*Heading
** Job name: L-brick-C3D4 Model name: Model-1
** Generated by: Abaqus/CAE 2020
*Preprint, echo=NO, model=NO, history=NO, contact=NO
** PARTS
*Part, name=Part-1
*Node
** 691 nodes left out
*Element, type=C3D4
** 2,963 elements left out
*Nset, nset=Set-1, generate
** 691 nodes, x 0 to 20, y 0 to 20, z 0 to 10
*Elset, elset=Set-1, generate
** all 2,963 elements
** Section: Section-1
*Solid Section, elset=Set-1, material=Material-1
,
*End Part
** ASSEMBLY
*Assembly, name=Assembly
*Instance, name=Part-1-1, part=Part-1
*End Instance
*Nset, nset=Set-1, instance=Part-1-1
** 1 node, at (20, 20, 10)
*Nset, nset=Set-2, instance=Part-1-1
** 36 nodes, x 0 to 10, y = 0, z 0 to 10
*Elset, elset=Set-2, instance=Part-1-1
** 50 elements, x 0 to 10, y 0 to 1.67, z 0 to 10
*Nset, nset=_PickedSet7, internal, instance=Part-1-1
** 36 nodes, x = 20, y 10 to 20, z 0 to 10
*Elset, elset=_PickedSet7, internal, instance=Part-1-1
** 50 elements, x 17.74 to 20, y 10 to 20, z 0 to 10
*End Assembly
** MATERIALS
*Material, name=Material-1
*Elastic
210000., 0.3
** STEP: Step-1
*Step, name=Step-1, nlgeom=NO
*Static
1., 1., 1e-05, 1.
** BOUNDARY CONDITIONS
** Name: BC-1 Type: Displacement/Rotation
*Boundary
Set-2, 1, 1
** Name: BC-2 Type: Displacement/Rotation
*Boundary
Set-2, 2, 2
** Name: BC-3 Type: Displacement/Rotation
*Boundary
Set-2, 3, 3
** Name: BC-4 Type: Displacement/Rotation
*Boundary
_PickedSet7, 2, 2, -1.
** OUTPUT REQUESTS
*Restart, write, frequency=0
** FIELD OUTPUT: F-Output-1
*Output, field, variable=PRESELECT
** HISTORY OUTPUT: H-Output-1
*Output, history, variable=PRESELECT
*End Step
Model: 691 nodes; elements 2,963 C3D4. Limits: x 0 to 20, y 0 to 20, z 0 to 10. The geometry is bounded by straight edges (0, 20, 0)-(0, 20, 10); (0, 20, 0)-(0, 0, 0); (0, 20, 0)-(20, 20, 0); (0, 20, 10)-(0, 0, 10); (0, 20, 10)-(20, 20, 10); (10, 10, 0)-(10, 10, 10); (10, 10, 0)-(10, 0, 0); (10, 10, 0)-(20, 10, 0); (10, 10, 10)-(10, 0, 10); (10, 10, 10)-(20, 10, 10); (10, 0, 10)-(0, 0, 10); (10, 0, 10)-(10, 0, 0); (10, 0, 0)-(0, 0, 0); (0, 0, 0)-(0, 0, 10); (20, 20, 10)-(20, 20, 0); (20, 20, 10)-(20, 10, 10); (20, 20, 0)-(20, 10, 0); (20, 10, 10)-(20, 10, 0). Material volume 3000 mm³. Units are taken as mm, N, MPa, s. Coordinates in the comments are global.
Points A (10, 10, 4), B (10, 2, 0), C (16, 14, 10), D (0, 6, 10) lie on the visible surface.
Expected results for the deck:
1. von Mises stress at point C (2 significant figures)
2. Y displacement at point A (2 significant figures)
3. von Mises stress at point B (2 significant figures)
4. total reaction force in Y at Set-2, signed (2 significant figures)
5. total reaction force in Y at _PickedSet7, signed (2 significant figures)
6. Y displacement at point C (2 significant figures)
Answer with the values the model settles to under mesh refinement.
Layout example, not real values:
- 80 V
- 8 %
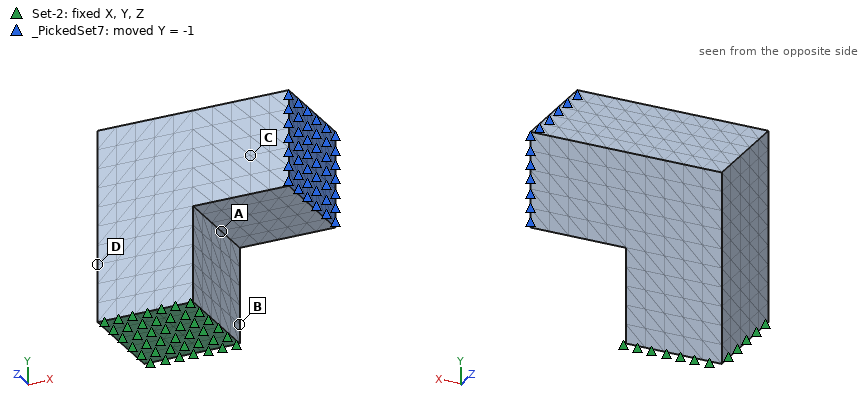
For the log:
- 1300 MPa
- -0.22 mm
- 3900 MPa
- 44000 N
- -44000 N
- -0.69 mm
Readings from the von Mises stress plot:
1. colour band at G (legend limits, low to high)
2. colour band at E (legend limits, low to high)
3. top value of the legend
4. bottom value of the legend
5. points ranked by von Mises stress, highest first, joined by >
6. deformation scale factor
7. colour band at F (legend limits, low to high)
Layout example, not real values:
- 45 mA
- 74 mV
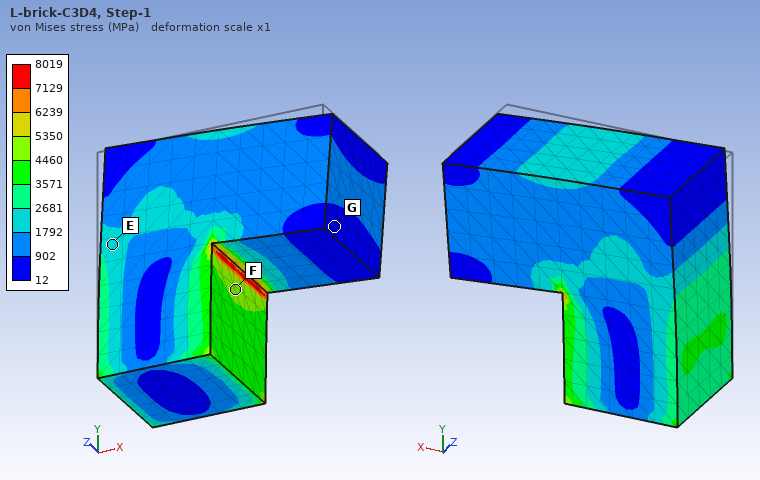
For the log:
- 12 to 902 MPa
- 1792 to 2681 MPa
- 8019 MPa
- 12 MPa
- F > E > G
- 1
- 4460 to 5350 MPa
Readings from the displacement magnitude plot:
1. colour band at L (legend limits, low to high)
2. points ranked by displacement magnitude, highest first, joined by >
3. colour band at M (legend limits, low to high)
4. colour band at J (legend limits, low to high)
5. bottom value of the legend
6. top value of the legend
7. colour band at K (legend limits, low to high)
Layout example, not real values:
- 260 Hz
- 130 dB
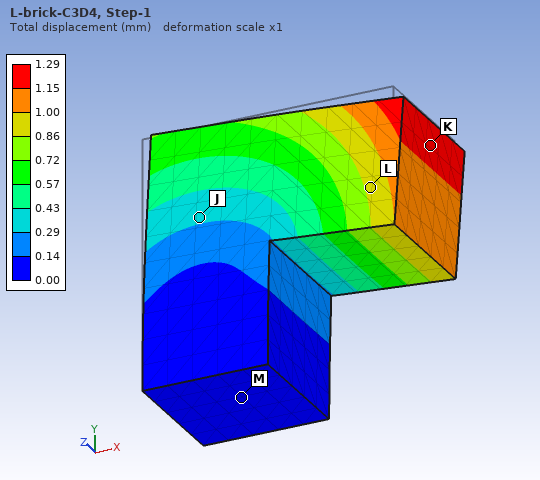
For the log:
- 0.86 to 1.00 mm
- K > L > J > M
- 0.00 to 0.14 mm
- 0.29 to 0.43 mm
- 0.00 mm
- 1.29 mm
- 1.15 to 1.29 mm
